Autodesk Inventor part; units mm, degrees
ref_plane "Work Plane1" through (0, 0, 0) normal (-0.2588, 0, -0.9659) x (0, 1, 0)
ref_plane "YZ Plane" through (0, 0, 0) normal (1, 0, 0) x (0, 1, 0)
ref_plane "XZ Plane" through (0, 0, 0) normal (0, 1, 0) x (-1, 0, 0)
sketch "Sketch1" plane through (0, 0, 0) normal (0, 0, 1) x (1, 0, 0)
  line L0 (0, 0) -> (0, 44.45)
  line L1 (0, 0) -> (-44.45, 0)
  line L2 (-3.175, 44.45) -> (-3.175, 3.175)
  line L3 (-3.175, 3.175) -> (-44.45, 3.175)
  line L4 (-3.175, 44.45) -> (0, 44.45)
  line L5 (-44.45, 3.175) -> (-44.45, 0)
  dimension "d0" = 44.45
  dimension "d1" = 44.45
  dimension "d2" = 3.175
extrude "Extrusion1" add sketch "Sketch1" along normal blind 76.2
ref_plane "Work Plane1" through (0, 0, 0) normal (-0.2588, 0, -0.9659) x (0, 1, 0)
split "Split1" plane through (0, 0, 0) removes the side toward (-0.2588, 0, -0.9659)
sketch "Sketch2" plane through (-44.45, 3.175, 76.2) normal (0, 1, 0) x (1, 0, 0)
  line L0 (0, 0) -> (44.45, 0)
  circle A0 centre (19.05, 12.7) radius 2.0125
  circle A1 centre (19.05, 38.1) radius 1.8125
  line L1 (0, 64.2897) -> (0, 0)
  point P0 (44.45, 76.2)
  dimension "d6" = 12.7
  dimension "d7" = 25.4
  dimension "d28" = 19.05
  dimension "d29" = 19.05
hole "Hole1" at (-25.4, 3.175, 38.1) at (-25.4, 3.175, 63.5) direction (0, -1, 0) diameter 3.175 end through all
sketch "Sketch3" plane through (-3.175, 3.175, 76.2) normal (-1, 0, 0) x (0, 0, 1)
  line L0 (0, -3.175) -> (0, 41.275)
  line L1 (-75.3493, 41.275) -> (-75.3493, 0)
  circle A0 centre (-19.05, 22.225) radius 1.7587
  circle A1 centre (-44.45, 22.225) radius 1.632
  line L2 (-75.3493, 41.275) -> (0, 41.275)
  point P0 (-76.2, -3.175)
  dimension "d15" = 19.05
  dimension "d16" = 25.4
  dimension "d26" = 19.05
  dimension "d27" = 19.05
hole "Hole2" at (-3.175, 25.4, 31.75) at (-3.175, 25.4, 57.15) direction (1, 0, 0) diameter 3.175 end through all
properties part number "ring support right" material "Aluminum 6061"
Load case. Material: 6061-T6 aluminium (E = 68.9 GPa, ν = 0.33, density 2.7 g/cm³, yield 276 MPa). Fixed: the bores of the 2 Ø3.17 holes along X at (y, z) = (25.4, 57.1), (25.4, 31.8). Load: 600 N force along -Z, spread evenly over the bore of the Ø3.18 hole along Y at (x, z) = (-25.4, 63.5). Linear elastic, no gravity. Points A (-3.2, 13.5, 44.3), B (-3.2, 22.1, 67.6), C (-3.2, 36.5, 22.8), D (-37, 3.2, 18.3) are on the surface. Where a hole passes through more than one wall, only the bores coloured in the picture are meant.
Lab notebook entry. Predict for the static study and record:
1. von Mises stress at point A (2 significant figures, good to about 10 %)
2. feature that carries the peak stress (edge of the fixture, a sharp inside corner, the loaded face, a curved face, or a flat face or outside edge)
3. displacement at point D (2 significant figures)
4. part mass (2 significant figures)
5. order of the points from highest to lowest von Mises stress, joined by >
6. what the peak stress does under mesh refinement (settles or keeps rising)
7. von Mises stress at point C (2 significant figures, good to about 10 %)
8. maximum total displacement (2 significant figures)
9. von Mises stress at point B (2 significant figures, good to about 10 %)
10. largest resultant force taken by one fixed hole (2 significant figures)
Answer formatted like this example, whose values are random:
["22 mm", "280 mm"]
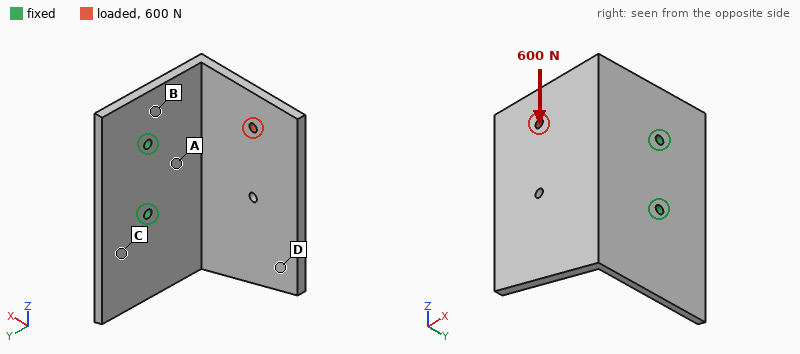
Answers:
["69 MPa", "edge of the fixture", "0.38 mm", "53 g", "A > B > C > D", "keeps rising", "34 MPa", "0.47 mm", "53 MPa", "740 N"]
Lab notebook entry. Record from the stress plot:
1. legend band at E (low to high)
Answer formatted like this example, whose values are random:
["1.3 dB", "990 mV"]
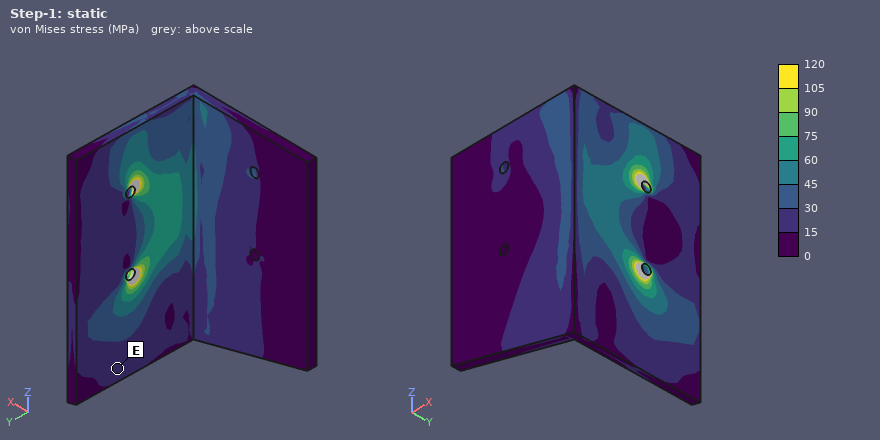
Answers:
["15 to 30 MPa"]
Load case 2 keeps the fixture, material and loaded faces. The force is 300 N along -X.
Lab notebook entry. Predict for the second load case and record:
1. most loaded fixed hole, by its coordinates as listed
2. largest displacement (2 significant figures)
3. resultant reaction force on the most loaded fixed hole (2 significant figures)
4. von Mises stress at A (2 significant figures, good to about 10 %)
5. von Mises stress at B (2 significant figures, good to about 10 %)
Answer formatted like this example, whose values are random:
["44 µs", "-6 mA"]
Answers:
["(25.4, 57.1)", "0.49 mm", "320 N", "40 MPa", "55 MPa"]
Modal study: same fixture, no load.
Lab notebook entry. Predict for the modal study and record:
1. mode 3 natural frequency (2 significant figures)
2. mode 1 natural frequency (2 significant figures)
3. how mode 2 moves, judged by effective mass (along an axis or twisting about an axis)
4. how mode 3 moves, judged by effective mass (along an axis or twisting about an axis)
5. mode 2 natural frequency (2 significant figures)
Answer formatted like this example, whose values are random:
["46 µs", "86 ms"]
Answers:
["2200 Hz", "730 Hz", "along Z", "along X", "1200 Hz"]
